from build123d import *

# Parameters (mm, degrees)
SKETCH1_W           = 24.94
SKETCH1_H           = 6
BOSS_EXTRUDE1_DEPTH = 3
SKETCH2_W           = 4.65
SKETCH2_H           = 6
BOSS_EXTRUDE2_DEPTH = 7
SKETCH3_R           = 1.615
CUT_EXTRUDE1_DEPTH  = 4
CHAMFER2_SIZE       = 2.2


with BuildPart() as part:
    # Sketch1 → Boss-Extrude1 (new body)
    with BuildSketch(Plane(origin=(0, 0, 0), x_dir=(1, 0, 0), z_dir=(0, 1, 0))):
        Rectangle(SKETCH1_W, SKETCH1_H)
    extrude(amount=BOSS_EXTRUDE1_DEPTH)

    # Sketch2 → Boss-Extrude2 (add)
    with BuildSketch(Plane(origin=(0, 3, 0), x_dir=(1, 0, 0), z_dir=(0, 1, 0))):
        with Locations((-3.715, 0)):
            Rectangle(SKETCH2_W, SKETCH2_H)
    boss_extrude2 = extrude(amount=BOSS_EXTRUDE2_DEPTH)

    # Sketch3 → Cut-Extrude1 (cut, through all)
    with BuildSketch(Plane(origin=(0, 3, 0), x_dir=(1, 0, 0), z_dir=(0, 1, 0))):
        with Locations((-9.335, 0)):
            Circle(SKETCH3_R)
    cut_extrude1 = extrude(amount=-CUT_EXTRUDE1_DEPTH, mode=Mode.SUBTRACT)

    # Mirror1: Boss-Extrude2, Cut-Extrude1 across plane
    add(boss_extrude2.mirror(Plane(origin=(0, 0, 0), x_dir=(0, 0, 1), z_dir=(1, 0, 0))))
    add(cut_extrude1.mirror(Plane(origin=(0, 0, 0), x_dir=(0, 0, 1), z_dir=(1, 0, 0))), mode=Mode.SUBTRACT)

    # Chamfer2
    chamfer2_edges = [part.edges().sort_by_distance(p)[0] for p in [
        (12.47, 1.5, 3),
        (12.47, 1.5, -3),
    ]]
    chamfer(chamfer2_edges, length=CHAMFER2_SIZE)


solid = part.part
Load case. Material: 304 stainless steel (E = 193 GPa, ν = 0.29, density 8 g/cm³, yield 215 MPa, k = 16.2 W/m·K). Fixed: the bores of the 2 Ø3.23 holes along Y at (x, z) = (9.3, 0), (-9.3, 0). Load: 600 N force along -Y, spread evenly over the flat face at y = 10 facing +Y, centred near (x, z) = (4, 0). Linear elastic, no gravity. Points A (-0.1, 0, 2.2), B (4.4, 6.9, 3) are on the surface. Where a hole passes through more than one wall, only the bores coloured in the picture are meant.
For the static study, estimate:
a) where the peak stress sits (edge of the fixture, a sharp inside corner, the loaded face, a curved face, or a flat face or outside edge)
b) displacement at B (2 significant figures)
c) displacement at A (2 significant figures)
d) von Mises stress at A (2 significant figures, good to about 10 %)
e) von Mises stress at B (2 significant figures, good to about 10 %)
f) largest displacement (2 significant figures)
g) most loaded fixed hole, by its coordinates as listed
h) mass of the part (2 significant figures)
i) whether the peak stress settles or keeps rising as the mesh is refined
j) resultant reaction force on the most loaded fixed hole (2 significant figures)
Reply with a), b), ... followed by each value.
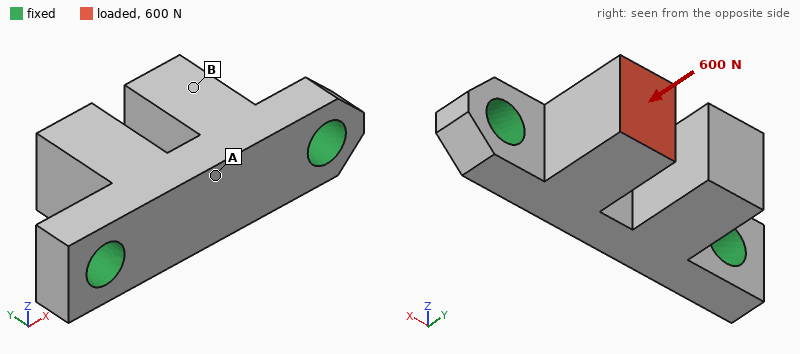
a) edge of the fixture
b) 4.2 µm
c) 3.9 µm
d) 52 MPa
e) 22 MPa
f) 6.9 µm
g) (9.3, 0)
h) 6.2 g
i) keeps rising
j) 470 N
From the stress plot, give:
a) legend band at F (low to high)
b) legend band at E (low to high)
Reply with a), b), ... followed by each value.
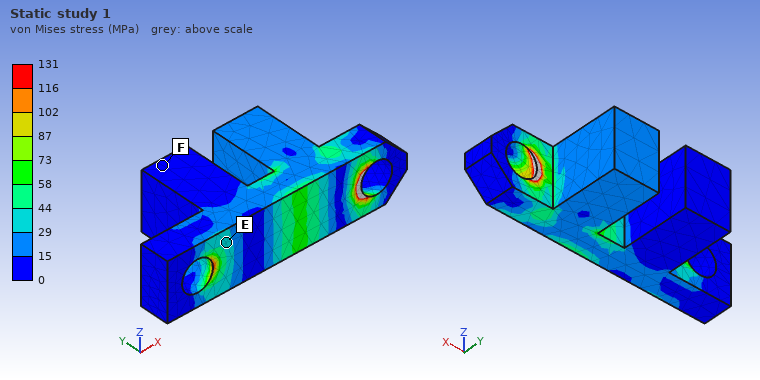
a) 0 to 15 MPa
b) 29 to 44 MPa
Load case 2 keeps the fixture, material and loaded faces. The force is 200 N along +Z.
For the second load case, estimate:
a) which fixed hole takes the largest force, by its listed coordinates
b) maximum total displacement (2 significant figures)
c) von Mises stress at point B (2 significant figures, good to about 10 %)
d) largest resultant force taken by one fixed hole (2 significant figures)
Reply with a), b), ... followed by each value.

a) (9.3, 0)
b) 13 µm
c) 23 MPa
d) 160 N
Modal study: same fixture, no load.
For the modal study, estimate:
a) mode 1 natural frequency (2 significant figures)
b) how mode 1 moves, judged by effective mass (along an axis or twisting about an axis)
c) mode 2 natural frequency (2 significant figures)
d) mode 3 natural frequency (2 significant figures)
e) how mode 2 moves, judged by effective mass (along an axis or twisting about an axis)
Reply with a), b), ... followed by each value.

a) 20 kHz
b) along Z
c) 22 kHz
d) 31 kHz
e) along Y
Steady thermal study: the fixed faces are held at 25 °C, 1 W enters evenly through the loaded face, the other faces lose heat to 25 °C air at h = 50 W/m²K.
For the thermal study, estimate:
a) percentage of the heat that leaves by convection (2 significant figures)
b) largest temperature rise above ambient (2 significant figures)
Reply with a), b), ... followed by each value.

a) 19 %
b) 23 K
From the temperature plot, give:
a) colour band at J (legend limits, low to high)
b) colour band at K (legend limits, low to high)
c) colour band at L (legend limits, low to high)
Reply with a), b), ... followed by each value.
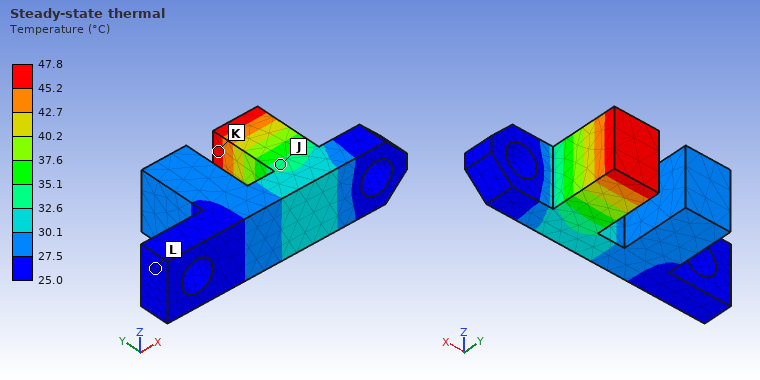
a) 32.6 to 35.1 °C
b) 45.2 to 47.8 °C
c) 25.0 to 27.5 °C
